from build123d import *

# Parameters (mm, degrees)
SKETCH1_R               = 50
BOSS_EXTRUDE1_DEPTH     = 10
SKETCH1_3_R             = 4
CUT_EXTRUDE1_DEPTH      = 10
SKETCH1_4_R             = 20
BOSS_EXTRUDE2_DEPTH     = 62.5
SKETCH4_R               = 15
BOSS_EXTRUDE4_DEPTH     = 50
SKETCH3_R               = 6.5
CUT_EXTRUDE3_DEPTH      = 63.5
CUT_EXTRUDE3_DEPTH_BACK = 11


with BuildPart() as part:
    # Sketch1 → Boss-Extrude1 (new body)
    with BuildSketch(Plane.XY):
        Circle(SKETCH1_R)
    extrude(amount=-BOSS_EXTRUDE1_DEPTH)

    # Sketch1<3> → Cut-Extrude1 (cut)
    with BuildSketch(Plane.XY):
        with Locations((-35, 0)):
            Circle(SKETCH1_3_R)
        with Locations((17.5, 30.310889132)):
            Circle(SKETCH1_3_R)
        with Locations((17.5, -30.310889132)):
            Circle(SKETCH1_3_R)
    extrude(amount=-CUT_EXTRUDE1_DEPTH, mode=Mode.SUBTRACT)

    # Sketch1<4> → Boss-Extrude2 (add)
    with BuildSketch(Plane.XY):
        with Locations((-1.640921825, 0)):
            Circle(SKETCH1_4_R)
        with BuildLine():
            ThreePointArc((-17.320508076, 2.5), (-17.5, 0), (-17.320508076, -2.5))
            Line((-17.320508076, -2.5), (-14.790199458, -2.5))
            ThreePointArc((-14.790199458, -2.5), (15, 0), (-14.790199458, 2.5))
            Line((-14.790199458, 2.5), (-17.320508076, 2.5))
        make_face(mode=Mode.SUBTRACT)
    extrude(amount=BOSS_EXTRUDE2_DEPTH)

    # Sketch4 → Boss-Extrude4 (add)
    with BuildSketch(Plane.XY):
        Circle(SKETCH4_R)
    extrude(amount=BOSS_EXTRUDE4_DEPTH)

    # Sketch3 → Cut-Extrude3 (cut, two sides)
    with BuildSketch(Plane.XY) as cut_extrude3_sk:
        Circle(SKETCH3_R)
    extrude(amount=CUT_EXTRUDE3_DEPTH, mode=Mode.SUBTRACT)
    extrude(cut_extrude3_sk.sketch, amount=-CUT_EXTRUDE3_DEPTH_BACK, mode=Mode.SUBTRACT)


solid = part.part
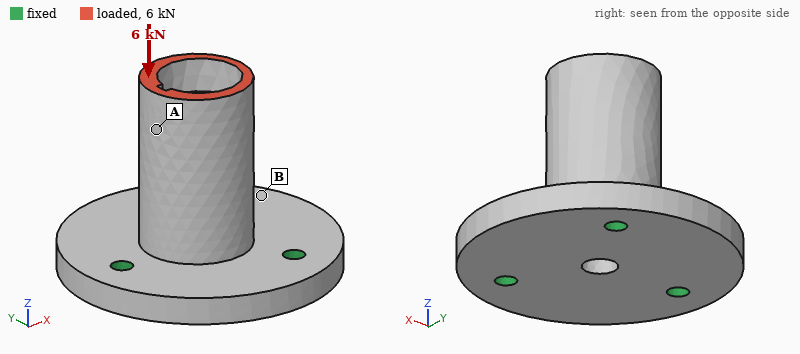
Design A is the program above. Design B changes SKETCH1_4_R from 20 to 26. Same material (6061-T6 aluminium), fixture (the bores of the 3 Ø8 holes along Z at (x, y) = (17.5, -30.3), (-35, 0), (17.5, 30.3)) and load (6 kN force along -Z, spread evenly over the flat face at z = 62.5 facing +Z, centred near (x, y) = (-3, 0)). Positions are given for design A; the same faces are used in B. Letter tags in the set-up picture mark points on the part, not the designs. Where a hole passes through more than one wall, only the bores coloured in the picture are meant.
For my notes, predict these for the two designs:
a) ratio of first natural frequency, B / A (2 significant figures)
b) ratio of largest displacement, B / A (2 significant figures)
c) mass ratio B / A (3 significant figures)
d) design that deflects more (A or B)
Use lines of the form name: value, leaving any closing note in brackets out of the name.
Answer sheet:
ratio of first natural frequency, B / A: 1.0
ratio of largest displacement, B / A: 0.47
mass ratio B / A: 1.39
design that deflects more: A
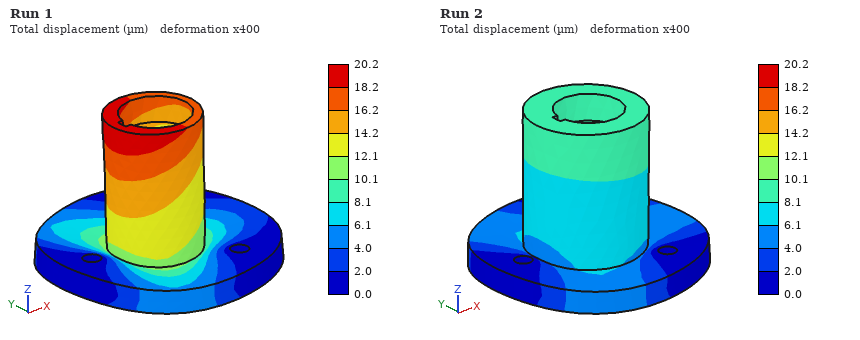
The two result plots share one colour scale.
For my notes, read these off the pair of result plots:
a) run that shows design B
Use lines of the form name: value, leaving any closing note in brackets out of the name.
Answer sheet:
run that shows design B: Run 2
